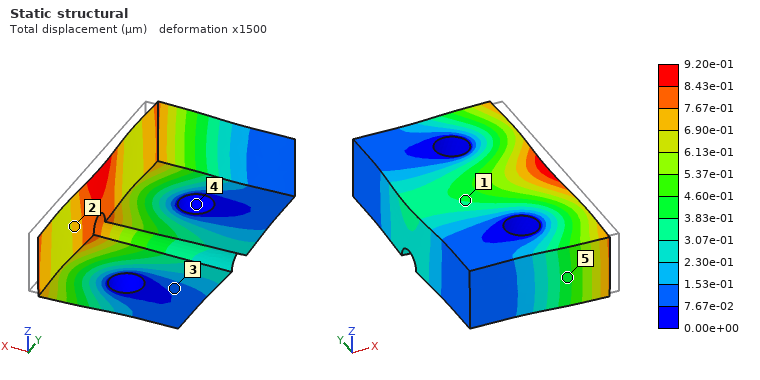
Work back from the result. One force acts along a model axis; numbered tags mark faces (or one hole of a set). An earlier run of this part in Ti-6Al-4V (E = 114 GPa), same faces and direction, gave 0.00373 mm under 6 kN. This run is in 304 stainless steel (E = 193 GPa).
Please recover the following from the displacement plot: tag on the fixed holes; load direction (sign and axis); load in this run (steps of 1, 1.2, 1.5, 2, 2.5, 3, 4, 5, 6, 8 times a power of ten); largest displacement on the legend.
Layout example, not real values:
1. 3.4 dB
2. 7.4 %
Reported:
1. 4
2. -X
3. 2.5 kN
4. 9.20e-01 µm
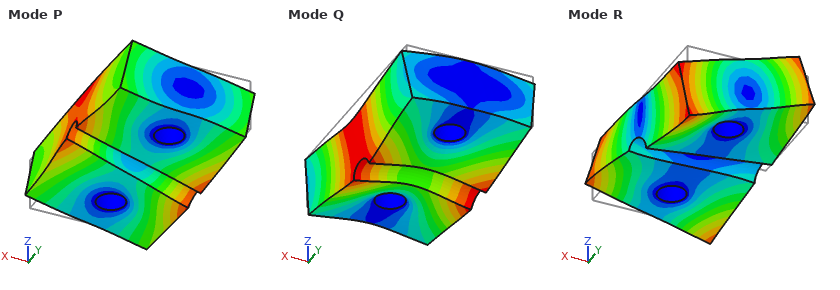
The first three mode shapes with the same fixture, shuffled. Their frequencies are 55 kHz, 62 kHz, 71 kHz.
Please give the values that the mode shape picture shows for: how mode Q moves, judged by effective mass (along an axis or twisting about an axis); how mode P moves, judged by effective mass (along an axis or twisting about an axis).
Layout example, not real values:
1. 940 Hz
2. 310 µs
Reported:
1. along Z
2. twisting about Y
